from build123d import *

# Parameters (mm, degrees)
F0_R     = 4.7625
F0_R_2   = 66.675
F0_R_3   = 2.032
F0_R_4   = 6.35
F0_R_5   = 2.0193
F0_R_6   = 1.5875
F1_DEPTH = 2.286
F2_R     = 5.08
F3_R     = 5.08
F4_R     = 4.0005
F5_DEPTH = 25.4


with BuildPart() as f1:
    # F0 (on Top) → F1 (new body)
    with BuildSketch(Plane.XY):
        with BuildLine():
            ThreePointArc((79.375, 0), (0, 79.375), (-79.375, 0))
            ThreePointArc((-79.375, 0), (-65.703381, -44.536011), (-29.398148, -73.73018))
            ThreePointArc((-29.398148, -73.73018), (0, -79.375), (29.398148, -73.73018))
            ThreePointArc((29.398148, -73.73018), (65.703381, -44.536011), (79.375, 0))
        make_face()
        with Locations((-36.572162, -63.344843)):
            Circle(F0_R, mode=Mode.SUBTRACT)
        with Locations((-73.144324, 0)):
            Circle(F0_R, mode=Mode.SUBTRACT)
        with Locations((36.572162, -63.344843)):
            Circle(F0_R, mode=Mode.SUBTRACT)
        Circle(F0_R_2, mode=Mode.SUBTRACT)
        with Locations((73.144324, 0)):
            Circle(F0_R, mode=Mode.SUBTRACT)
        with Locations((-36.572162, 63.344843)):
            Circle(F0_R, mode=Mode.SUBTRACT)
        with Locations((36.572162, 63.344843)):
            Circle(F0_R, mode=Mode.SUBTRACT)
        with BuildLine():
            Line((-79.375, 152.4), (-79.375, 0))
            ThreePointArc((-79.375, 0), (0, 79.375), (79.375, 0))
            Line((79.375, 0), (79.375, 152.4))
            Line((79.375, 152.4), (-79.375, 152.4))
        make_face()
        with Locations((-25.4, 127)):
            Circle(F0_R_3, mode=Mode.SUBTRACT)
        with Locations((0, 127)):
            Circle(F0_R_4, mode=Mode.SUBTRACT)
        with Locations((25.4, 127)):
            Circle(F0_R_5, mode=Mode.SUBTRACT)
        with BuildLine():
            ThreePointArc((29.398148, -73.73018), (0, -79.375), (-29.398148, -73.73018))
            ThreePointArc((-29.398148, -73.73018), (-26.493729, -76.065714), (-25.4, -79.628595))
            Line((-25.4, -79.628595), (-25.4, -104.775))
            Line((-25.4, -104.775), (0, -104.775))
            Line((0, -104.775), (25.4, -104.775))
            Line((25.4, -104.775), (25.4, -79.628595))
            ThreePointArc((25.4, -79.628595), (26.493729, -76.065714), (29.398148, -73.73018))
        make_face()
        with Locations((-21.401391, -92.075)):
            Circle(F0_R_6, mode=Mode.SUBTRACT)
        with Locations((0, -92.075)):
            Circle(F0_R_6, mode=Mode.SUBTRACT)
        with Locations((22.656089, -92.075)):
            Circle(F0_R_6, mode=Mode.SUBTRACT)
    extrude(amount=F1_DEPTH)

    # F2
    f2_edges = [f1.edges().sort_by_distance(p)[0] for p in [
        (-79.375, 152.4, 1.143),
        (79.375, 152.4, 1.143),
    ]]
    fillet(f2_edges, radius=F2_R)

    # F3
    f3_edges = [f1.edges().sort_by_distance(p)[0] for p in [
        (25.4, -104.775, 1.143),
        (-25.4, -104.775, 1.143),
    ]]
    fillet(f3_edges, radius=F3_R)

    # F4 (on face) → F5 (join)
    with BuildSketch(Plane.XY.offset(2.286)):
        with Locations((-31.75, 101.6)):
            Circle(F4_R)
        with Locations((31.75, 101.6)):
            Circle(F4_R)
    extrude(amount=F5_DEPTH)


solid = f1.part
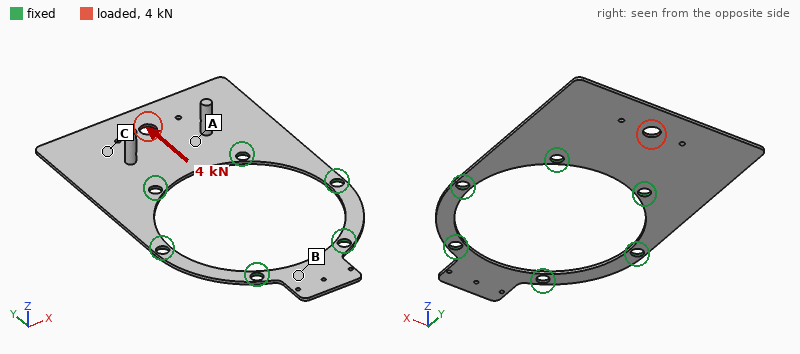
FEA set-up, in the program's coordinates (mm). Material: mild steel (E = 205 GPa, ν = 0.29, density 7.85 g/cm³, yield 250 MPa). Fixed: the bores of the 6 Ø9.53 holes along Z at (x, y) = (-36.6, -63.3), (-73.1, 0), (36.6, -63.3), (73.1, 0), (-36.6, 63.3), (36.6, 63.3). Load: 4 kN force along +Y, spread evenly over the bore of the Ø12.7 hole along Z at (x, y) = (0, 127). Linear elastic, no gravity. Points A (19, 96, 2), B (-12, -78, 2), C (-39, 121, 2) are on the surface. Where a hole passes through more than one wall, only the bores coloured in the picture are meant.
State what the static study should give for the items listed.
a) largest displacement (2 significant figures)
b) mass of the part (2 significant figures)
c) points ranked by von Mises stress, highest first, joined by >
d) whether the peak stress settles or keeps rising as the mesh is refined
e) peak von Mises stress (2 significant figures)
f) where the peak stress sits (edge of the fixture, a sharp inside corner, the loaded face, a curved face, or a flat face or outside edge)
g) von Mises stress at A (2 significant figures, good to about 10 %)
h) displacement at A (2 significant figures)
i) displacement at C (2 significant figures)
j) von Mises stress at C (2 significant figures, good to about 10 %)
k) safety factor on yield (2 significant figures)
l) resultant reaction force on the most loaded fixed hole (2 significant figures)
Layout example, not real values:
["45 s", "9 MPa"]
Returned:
["13 µm", "390 g", "A > C > B", "settles", "86 MPa", "the loaded face", "24 MPa", "5.4 µm", "4.4 µm", "9.8 MPa", "2.9", "1.9 kN"]
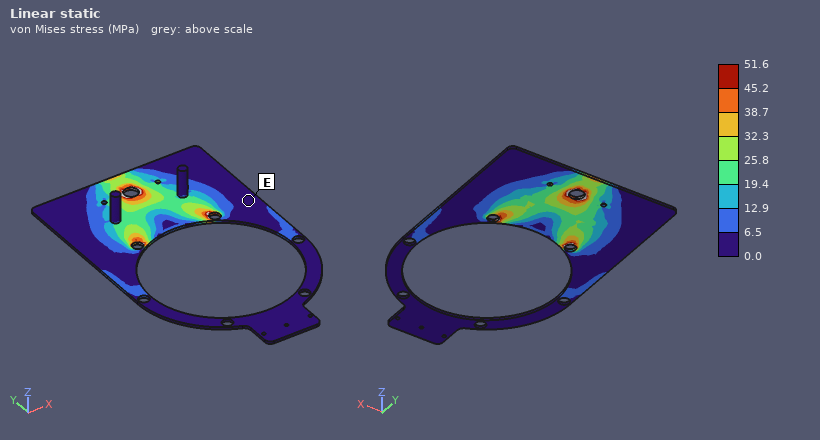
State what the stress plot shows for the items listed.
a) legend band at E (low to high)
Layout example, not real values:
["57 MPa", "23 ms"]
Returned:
["0.0 to 6.5 MPa"]
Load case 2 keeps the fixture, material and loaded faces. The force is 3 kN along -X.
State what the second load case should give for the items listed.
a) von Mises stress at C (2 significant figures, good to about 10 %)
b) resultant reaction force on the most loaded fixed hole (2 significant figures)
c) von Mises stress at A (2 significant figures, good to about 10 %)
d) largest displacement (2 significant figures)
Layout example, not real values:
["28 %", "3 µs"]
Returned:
["11 MPa", "1.9 kN", "23 MPa", "19 µm"]
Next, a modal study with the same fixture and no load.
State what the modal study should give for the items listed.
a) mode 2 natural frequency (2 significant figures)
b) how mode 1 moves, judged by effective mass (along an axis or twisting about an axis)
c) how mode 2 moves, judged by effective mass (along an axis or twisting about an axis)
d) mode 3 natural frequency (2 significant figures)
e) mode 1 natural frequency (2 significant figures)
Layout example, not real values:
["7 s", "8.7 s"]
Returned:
["360 Hz", "along Z", "twisting about Y", "670 Hz", "220 Hz"]
